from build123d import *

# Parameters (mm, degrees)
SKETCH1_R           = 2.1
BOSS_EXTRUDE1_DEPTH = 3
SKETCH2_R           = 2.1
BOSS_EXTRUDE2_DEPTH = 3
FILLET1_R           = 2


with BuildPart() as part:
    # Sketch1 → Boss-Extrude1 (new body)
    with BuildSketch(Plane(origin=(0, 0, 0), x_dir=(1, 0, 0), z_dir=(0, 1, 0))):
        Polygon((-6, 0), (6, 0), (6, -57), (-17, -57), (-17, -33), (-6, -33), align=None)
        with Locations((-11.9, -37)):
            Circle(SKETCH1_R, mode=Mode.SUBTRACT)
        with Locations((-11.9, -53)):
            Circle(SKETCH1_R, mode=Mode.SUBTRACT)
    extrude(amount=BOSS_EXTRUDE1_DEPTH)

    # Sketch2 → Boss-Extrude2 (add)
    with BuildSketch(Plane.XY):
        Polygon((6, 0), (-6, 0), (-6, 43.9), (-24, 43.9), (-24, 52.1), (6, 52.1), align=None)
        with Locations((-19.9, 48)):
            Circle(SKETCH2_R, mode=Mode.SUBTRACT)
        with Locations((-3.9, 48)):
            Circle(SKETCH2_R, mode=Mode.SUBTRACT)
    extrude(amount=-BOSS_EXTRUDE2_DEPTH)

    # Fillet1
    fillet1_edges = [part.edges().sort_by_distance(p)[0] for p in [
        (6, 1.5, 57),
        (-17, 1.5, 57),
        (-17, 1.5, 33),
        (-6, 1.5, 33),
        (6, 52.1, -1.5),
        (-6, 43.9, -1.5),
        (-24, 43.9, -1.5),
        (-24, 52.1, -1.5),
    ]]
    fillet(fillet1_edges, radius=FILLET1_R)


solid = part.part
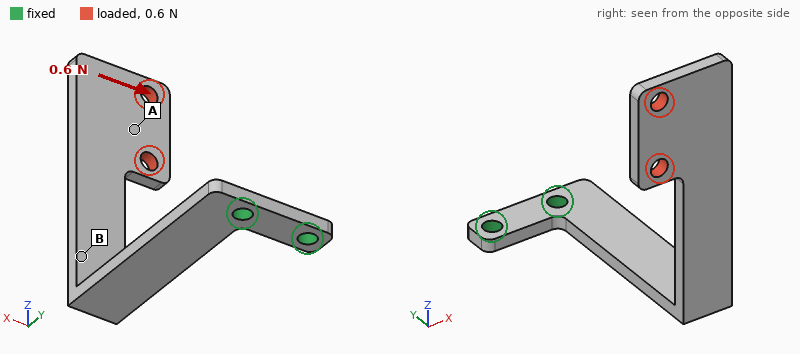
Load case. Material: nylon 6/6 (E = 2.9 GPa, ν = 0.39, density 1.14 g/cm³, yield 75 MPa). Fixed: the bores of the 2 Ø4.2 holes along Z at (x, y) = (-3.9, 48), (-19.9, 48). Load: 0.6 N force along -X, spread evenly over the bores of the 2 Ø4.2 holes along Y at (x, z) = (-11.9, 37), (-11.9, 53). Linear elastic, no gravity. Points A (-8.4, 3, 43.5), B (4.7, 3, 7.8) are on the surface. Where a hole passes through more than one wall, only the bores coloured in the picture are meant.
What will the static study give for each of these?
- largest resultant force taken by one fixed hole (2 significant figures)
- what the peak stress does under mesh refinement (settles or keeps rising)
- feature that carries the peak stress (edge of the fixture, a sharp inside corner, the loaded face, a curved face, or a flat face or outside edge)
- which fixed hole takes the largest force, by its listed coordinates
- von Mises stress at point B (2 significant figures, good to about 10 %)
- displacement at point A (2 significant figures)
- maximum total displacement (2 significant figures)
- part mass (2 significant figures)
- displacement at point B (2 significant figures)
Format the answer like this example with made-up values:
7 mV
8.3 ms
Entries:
0.72 N
keeps rising
edge of the fixture
(-19.9, 48)
0.29 MPa
0.62 mm
0.81 mm
5.7 g
0.16 mm
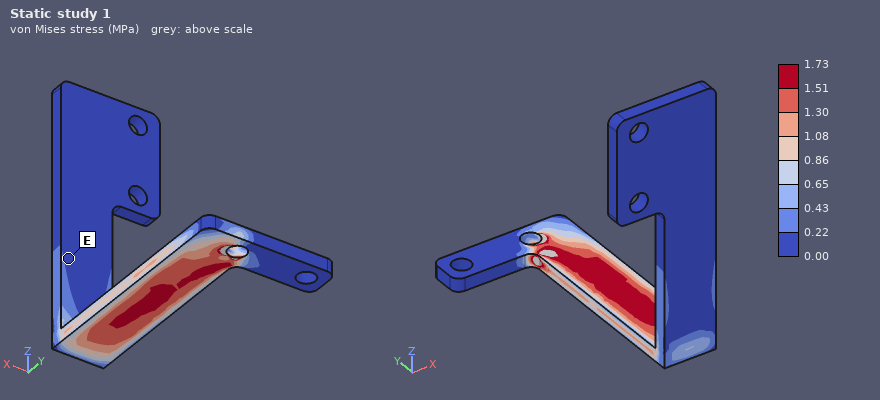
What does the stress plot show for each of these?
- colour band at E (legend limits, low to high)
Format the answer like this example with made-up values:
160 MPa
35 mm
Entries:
0.00 to 0.22 MPa
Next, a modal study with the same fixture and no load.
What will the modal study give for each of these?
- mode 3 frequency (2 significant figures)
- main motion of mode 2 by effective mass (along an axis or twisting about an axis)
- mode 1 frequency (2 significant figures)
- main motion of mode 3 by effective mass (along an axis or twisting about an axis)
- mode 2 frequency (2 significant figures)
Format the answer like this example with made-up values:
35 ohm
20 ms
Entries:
220 Hz
along X
76 Hz
along Z
110 Hz
